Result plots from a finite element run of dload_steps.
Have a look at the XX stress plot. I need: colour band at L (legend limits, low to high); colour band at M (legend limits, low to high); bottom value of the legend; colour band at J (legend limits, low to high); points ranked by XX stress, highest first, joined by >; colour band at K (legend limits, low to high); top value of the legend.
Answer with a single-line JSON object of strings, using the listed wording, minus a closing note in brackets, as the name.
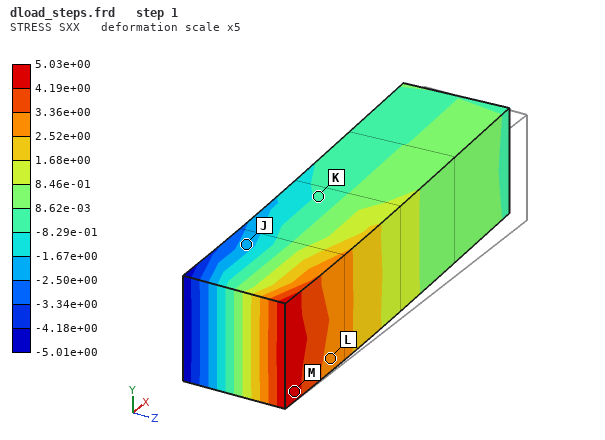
{"colour band at L": "2.52e+00 to 3.36e+00", "colour band at M": "4.19e+00 to 5.03e+00", "bottom value of the legend": "-5.01e+00", "colour band at J": "-2.50e+00 to -1.67e+00", "points ranked by XX stress, highest first, joined by >": "M > L > K > J", "colour band at K": "-8.29e-01 to 8.62e-03", "top value of the legend": "5.03e+00"}
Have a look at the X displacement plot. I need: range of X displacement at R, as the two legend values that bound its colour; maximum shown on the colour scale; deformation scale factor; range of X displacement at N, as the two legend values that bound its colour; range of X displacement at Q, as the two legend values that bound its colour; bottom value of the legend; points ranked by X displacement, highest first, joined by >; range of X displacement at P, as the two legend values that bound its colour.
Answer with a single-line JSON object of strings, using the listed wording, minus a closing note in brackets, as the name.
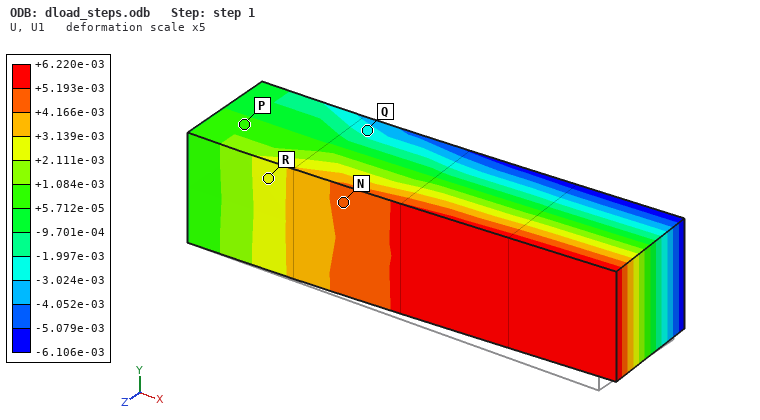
{"range of X displacement at R, as the two legend values that bound its colour": "+2.111e-03 to +3.139e-03", "maximum shown on the colour scale": "+6.220e-03", "deformation scale factor": "5", "range of X displacement at N, as the two legend values that bound its colour": "+4.166e-03 to +5.193e-03", "range of X displacement at Q, as the two legend values that bound its colour": "-3.024e-03 to -1.997e-03", "bottom value of the legend": "-6.106e-03", "points ranked by X displacement, highest first, joined by >": "N > R > P > Q", "range of X displacement at P, as the two legend values that bound its colour": "+5.712e-05 to +1.084e-03"}
